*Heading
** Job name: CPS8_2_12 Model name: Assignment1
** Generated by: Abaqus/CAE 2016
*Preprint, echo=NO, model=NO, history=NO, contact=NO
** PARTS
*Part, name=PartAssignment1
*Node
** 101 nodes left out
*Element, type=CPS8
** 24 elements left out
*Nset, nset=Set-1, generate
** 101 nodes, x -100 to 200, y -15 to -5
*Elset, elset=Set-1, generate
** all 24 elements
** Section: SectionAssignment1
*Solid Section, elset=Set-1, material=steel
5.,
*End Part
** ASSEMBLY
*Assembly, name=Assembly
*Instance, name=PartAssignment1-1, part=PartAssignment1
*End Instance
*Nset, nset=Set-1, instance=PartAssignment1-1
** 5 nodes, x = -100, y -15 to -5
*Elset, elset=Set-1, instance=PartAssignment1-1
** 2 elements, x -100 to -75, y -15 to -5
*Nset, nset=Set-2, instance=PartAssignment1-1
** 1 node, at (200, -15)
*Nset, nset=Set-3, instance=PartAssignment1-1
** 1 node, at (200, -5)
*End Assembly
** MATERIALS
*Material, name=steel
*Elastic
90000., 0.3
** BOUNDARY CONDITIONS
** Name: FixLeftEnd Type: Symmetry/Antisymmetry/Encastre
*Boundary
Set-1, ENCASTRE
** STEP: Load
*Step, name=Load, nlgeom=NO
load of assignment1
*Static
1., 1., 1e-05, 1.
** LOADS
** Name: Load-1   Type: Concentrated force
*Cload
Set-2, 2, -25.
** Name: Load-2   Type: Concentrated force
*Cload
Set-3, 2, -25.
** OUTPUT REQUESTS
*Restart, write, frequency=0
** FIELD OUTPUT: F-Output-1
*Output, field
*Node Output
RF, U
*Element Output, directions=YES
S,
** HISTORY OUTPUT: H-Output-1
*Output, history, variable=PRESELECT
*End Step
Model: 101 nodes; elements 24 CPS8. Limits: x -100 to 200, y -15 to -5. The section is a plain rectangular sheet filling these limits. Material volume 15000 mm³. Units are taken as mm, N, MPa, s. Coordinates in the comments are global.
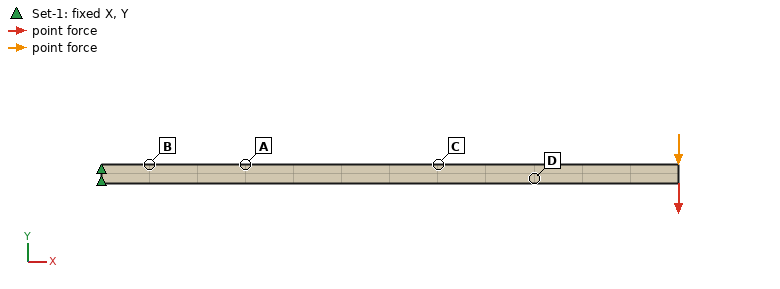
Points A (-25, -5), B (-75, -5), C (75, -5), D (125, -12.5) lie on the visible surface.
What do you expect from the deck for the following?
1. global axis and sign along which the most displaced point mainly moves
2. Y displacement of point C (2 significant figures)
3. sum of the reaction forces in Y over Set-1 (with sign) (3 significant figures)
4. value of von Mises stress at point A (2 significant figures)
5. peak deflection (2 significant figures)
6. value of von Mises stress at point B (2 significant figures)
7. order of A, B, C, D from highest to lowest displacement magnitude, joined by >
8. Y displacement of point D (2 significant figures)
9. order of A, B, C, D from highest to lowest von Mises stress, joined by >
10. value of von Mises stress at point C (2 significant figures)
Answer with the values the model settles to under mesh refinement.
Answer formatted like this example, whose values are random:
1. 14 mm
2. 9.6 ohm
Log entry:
1. -Y
2. -4.9 mm
3. 50.0 N
4. 130 MPa
5. 12 mm
6. 160 MPa
7. D > C > A > B
8. -7.5 mm
9. B > A > C > D
10. 74 MPa
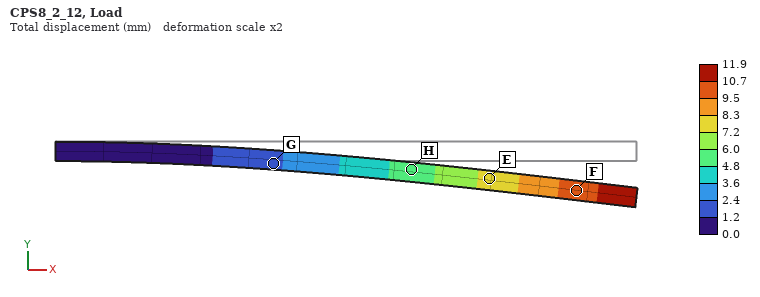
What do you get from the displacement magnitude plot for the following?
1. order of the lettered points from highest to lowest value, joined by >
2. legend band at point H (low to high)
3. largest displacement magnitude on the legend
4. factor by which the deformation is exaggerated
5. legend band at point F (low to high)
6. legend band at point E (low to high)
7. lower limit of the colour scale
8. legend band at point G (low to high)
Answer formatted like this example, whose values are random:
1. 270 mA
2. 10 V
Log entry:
1. F > E > H > G
2. 4.8 to 6.0 mm
3. 11.9 mm
4. 2
5. 9.5 to 10.7 mm
6. 7.2 to 8.3 mm
7. 0.0 mm
8. 1.2 to 2.4 mm
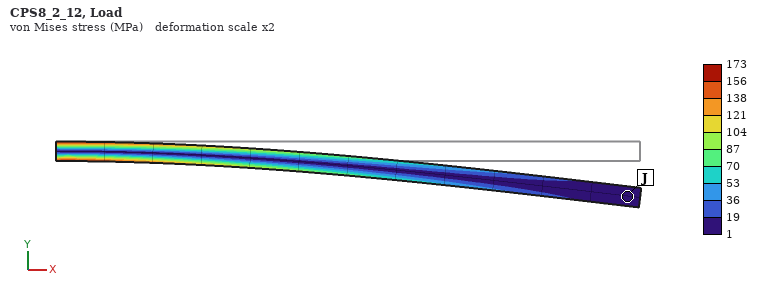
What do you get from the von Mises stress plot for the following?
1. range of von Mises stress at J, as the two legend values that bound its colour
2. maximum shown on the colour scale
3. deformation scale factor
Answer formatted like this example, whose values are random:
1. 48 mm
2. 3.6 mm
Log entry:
1. 1 to 19 MPa
2. 173 MPa
3. 2
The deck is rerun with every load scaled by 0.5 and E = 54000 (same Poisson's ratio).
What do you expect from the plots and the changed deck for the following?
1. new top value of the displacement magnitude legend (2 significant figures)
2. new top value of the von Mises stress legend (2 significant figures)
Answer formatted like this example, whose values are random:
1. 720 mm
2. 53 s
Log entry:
1. 9.9 mm
2. 86 MPa
